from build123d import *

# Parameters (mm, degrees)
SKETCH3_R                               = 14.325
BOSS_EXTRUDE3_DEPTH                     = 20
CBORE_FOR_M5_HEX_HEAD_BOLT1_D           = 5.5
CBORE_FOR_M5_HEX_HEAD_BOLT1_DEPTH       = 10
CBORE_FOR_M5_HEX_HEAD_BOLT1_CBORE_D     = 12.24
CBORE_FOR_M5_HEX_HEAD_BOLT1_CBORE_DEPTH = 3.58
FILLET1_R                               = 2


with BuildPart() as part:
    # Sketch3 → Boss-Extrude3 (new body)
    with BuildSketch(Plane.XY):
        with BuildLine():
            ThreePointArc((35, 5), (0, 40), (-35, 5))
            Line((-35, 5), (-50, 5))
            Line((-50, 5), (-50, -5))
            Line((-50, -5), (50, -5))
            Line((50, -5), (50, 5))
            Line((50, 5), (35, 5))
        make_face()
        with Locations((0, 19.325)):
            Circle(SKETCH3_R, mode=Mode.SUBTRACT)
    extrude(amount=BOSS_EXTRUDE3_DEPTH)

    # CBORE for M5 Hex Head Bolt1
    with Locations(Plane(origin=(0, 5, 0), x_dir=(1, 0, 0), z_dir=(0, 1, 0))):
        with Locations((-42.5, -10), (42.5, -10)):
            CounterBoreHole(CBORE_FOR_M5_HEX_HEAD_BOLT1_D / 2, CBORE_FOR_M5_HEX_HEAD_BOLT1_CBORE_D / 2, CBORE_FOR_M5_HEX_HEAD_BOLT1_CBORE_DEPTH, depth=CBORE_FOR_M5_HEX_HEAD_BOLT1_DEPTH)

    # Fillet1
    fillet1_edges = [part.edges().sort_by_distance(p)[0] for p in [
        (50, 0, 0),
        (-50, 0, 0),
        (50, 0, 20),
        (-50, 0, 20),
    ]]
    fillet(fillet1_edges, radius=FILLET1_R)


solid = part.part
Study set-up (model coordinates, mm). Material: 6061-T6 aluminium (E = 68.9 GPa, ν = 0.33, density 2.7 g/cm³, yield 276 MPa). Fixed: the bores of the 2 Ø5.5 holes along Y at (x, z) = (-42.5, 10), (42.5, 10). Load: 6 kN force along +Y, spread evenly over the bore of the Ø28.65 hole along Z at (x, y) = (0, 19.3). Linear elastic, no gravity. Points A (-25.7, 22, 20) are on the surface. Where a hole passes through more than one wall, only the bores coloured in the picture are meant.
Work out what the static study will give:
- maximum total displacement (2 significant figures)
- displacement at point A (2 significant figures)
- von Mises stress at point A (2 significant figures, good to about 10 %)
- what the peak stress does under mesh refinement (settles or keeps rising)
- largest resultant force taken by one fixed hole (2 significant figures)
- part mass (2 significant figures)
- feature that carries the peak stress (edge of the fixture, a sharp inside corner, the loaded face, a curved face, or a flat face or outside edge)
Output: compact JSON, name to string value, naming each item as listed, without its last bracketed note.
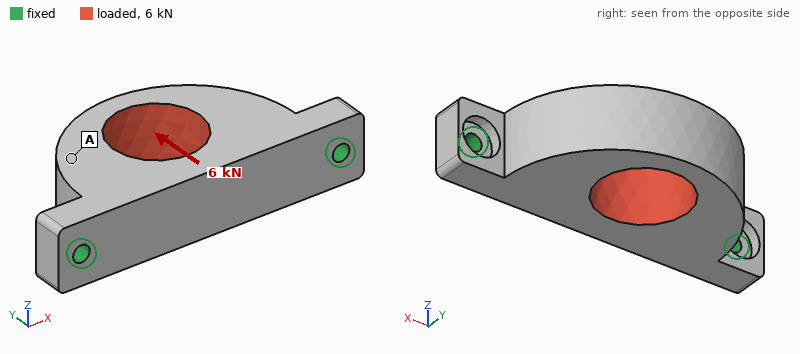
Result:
{"maximum total displacement": "33 µm", "displacement at point A": "24 µm", "von Mises stress at point A": "16 MPa", "what the peak stress does under mesh refinement": "keeps rising", "largest resultant force taken by one fixed hole": "3.5 kN", "part mass": "120 g", "feature that carries the peak stress": "edge of the fixture"}
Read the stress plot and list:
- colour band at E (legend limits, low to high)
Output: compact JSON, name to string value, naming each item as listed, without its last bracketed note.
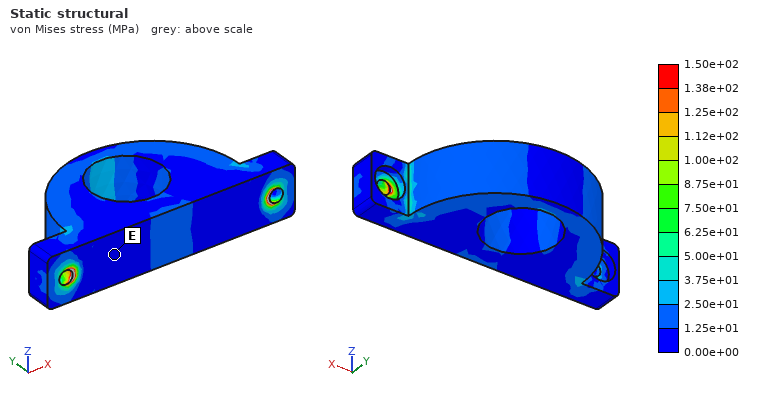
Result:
{"colour band at E": "0.00e+00 to 1.25e+01 MPa"}
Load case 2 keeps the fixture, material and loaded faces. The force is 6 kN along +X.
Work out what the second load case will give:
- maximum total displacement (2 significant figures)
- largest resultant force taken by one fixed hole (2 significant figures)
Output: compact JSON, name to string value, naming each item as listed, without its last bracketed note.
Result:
{"maximum total displacement": "25 µm", "largest resultant force taken by one fixed hole": "3.4 kN"}
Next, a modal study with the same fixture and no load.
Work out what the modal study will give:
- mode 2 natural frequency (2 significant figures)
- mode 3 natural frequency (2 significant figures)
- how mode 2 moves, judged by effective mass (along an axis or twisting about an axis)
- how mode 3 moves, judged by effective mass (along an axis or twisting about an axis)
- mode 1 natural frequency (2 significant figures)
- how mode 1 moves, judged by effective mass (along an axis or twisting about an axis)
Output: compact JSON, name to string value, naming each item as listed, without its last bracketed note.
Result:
{"mode 2 natural frequency": "7600 Hz", "mode 3 natural frequency": "8200 Hz", "how mode 2 moves, judged by effective mass": "along Y", "how mode 3 moves, judged by effective mass": "along Z", "mode 1 natural frequency": "2700 Hz", "how mode 1 moves, judged by effective mass": "along Z"}
